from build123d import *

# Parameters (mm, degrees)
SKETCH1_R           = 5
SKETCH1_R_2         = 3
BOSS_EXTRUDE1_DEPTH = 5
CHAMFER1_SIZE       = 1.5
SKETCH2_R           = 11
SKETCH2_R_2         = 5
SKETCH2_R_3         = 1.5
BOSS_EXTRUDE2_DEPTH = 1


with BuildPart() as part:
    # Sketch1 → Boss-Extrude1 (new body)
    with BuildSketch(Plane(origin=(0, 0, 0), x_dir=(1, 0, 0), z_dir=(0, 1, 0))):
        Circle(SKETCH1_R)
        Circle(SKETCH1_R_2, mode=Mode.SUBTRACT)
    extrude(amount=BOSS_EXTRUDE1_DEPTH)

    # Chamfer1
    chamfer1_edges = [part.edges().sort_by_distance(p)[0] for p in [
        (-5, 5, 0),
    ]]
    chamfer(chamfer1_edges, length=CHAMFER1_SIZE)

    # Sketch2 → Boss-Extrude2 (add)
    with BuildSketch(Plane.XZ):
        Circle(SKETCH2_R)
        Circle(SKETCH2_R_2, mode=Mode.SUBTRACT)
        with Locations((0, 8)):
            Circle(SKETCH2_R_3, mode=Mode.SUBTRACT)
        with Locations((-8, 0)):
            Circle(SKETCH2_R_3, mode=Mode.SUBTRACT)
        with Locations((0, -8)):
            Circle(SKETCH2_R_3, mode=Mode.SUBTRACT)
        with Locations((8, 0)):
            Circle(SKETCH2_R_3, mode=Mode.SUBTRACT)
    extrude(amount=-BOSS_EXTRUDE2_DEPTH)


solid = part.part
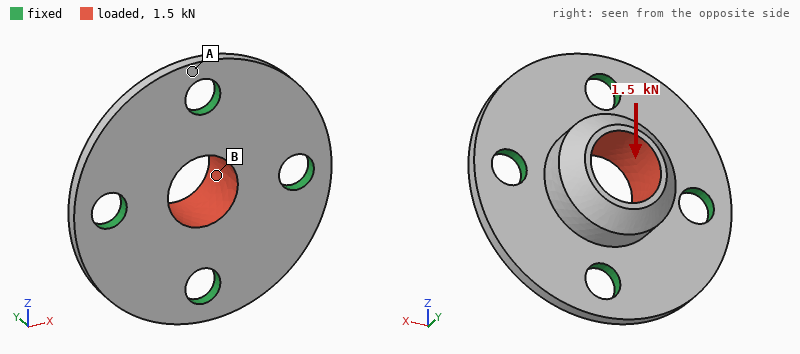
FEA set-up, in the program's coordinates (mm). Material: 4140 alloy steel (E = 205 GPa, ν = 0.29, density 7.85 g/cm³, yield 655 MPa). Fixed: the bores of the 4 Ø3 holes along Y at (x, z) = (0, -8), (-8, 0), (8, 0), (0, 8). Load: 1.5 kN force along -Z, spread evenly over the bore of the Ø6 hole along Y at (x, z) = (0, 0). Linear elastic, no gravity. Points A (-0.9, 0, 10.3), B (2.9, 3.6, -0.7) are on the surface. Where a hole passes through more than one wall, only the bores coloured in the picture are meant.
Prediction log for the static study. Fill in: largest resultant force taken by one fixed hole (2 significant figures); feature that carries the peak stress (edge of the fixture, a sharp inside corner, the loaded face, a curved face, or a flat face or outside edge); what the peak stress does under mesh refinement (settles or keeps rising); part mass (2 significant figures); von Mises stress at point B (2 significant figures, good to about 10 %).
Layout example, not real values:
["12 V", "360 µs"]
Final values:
["530 N", "edge of the fixture", "keeps rising", "3.9 g", "59 MPa"]
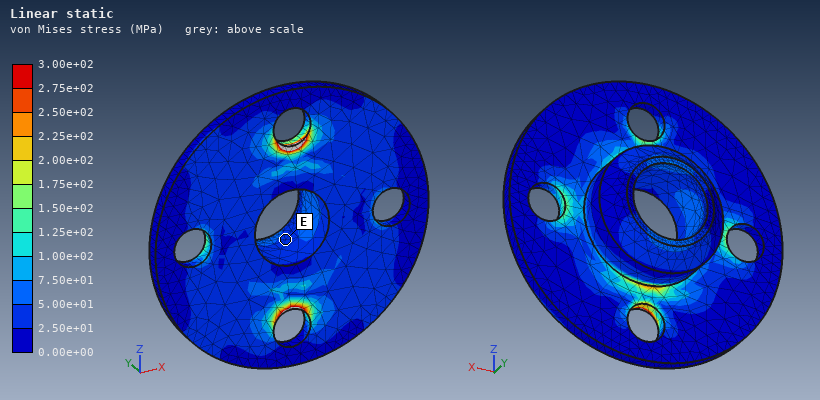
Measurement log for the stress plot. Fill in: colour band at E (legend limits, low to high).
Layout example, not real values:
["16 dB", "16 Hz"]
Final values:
["2.50e+01 to 5.00e+01 MPa"]
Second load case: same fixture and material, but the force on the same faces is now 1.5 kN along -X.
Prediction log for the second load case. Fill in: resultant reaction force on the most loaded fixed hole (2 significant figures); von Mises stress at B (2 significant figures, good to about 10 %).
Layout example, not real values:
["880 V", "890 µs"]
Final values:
["530 N", "44 MPa"]
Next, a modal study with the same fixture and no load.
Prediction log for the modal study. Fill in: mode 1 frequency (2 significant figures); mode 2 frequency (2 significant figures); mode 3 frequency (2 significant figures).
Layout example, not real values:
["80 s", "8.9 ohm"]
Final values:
["37 kHz", "37 kHz", "37 kHz"]
